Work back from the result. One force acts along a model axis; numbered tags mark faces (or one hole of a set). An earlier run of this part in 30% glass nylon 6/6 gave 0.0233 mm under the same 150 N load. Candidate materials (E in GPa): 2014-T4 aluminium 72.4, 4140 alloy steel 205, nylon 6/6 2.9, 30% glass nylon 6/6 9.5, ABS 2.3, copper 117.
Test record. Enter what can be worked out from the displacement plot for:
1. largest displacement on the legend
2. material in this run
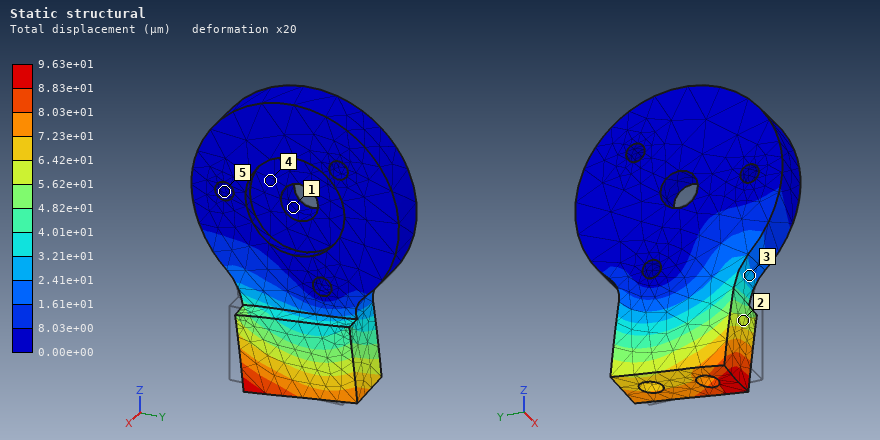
9.63e+01 µm
ABS
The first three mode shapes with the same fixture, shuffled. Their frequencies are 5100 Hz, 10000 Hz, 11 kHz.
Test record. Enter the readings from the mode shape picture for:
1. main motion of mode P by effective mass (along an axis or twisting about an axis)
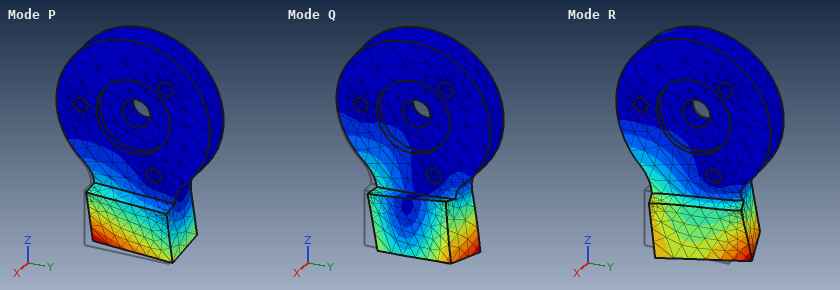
along X
